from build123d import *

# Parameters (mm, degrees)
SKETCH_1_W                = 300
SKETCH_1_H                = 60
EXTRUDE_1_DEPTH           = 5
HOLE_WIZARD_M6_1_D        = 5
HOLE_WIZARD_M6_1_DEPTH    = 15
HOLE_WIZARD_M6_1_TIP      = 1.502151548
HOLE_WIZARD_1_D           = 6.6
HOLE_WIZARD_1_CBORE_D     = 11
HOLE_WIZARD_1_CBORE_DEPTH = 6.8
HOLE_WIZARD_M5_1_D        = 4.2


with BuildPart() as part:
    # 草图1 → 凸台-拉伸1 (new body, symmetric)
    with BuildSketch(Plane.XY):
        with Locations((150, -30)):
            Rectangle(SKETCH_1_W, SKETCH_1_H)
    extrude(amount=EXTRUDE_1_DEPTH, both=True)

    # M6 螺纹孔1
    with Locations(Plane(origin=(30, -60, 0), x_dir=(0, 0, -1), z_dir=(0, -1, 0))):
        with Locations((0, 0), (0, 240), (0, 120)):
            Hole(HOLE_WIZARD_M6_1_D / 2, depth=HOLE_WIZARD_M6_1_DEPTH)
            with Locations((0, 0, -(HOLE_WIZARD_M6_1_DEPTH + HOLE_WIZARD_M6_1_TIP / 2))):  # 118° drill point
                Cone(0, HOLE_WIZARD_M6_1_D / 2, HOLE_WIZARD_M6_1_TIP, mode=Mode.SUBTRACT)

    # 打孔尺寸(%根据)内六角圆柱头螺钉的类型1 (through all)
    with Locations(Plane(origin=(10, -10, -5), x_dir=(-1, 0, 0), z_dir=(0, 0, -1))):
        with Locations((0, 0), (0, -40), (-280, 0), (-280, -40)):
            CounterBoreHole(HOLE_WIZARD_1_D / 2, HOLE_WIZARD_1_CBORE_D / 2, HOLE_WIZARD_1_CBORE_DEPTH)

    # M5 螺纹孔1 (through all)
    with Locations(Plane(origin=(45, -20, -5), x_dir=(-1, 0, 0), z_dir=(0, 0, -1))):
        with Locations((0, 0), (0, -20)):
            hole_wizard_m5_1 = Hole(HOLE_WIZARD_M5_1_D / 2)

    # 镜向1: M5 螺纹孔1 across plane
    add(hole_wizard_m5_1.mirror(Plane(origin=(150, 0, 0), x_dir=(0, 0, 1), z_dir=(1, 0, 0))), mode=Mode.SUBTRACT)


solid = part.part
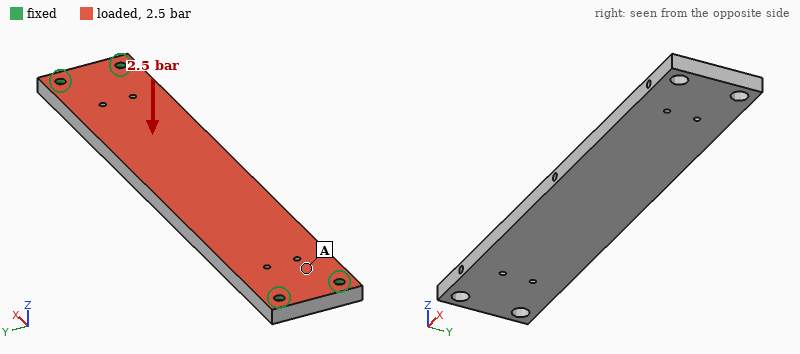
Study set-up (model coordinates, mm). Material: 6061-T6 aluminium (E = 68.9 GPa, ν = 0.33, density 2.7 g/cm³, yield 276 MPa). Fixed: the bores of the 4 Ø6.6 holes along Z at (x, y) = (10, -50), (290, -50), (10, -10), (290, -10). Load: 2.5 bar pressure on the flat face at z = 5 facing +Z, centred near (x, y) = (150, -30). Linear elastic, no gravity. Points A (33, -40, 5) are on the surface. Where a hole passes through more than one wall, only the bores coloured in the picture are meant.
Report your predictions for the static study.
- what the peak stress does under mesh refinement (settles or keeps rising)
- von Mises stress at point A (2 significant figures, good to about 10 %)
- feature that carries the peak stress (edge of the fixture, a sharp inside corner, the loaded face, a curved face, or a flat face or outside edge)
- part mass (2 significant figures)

keeps rising
46 MPa
edge of the fixture
470 g
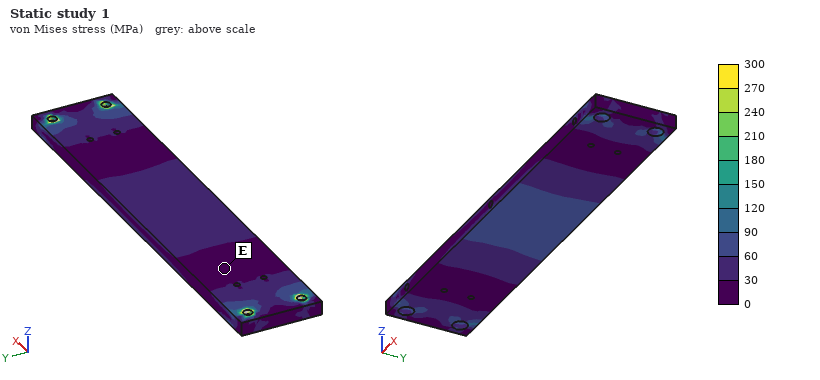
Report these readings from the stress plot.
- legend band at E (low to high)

0 to 30 MPa
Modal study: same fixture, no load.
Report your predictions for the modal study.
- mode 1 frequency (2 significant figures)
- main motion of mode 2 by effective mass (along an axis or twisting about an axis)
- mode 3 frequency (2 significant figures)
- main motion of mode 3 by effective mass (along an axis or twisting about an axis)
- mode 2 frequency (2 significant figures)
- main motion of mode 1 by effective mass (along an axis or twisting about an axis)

530 Hz
twisting about Y
1800 Hz
twisting about X
1500 Hz
along Z
